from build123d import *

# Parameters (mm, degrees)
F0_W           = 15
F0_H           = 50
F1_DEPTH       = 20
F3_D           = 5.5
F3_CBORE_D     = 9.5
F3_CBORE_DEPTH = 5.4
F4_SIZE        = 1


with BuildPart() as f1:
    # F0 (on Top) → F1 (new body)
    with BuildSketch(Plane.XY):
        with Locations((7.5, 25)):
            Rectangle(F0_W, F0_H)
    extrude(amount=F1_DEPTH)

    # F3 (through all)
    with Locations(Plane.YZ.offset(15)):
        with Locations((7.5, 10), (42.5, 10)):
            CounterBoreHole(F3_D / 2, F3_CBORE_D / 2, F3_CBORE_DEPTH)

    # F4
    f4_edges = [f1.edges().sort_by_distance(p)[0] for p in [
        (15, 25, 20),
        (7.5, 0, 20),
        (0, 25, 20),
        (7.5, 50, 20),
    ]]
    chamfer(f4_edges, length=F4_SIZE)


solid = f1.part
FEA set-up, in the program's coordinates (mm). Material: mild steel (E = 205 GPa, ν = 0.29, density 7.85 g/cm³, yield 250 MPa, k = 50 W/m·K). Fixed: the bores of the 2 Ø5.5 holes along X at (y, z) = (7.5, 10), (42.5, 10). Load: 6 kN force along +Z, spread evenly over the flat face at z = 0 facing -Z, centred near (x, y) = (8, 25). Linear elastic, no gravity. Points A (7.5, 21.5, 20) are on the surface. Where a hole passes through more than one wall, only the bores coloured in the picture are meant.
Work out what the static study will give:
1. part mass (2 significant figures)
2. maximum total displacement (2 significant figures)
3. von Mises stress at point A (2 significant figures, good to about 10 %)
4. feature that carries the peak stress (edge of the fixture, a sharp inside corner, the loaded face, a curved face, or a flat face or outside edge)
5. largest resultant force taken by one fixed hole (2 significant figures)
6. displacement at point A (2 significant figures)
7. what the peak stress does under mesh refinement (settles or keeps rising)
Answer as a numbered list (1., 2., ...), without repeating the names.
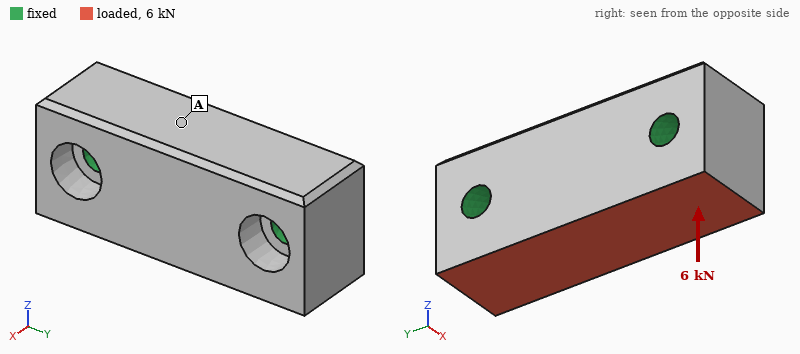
1. 110 g
2. 3.0 µm
3. 12 MPa
4. edge of the fixture
5. 3.0 kN
6. 1.8 µm
7. keeps rising
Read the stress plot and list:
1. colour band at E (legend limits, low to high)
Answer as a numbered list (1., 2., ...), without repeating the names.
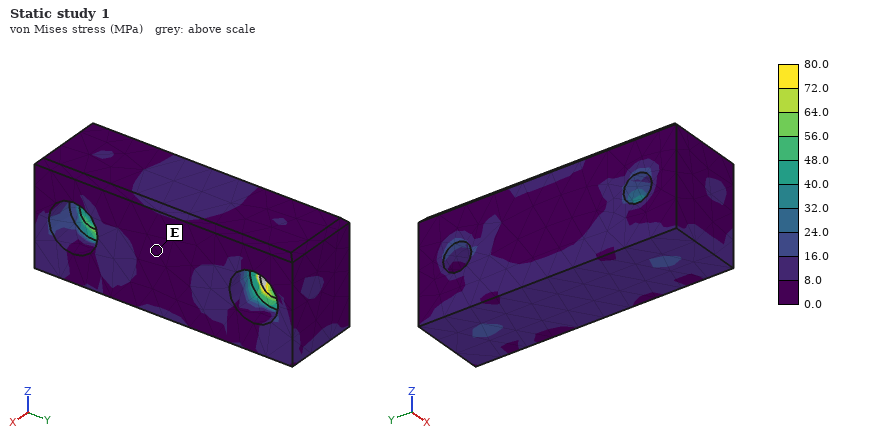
1. 0.0 to 8.0 MPa
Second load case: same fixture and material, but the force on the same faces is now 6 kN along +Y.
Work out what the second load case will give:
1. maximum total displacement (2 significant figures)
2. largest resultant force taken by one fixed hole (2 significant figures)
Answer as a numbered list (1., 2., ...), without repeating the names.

1. 2.9 µm
2. 3.3 kN
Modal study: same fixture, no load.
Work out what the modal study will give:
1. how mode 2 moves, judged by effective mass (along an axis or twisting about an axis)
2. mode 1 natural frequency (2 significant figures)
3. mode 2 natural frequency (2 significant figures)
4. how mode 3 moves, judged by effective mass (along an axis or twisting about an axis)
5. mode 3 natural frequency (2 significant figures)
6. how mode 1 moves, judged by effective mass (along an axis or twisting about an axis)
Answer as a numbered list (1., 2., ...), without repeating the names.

1. along X
2. 25 kHz
3. 29 kHz
4. along Z
5. 33 kHz
6. along Z
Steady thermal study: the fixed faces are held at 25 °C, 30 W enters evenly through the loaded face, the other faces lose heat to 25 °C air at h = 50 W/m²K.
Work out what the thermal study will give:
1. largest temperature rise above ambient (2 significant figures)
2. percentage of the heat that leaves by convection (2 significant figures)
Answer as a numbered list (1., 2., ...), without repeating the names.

1. 15 K
2. 3.2 %
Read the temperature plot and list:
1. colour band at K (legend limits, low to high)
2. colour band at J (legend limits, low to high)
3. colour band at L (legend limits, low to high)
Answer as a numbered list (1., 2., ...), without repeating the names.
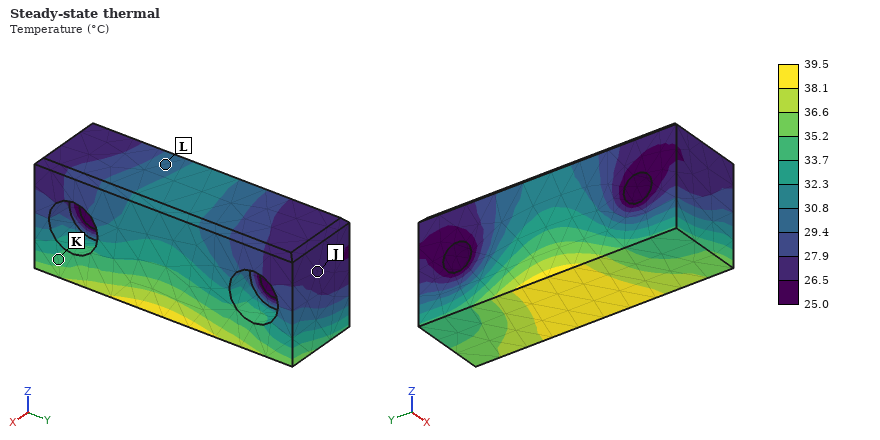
1. 33.7 to 35.2 °C
2. 26.5 to 27.9 °C
3. 29.4 to 30.8 °C
